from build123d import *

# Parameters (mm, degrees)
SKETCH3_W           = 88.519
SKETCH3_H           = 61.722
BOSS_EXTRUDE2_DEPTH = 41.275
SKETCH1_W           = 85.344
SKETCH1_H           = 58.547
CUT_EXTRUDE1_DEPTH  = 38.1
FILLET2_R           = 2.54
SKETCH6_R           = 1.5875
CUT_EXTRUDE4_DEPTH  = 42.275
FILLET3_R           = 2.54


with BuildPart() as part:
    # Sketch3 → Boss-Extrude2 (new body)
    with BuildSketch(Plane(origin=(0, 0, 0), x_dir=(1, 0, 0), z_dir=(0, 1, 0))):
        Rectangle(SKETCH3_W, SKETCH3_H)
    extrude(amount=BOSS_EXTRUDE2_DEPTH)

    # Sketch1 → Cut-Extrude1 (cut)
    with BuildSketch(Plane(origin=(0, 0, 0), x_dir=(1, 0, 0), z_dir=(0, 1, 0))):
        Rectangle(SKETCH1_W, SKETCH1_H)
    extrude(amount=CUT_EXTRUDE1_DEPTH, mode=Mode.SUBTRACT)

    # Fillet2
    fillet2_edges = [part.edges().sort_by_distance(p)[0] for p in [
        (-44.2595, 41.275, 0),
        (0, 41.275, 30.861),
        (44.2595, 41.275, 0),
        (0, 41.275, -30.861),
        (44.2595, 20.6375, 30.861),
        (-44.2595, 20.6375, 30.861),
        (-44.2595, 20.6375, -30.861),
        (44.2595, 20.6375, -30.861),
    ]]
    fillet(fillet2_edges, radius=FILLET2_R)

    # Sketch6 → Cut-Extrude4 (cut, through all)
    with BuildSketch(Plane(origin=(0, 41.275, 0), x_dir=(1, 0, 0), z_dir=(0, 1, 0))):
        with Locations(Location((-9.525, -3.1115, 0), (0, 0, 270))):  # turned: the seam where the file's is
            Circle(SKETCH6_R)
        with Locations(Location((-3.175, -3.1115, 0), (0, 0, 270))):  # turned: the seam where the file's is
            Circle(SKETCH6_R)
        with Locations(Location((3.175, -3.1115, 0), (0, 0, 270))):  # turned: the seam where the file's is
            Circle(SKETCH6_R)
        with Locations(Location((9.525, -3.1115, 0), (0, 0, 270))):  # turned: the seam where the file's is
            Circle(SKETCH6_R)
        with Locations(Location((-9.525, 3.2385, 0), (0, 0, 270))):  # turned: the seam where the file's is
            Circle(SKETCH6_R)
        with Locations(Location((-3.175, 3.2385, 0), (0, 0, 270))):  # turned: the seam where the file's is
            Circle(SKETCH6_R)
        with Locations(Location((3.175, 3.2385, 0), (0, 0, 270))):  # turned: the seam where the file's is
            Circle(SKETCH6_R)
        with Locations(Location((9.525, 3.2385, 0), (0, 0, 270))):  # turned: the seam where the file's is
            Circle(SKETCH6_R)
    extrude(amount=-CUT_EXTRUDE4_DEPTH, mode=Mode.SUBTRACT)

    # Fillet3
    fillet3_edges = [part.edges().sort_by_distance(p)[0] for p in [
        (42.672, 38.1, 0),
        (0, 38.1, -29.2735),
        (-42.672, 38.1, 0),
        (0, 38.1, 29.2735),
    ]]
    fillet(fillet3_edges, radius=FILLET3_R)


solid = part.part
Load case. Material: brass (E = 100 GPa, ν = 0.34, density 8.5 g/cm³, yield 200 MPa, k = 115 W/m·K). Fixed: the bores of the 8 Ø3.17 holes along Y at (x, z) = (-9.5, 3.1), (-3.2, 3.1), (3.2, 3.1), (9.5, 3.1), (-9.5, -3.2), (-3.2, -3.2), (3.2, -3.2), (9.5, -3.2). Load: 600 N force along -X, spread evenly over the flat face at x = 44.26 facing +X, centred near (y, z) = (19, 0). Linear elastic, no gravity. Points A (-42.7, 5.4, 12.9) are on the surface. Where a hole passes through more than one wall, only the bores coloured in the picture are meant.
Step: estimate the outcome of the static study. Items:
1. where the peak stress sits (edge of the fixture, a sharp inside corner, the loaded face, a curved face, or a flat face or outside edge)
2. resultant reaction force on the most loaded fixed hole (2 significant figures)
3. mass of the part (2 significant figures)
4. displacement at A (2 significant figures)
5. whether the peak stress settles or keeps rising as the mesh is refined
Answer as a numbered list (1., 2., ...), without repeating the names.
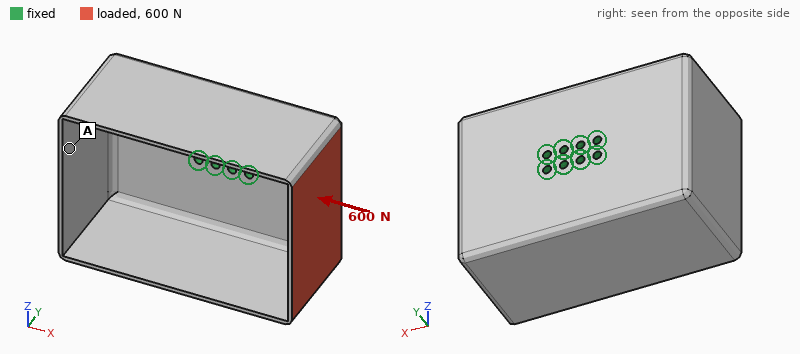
1. edge of the fixture
2. 250 N
3. 290 g
4. 0.13 mm
5. keeps rising
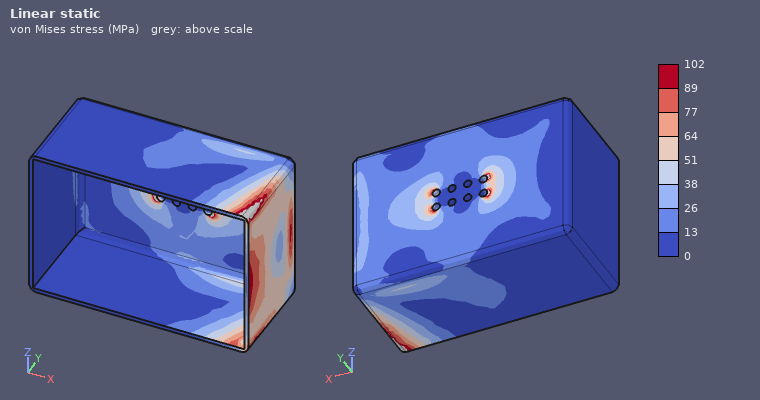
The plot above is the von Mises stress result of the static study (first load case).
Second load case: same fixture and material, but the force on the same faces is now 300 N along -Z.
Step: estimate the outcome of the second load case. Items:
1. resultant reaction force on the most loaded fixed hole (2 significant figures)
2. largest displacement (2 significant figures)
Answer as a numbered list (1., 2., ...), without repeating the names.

1. 430 N
2. 0.23 mm
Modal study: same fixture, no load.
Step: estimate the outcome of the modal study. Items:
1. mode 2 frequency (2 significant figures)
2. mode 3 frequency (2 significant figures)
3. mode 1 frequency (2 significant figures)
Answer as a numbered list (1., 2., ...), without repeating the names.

1. 640 Hz
2. 640 Hz
3. 610 Hz
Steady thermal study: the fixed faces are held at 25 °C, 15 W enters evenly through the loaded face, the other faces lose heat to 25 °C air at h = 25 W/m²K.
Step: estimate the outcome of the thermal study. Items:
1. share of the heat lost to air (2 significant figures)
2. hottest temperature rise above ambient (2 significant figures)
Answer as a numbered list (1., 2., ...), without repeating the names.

1. 36 %
2. 29 K
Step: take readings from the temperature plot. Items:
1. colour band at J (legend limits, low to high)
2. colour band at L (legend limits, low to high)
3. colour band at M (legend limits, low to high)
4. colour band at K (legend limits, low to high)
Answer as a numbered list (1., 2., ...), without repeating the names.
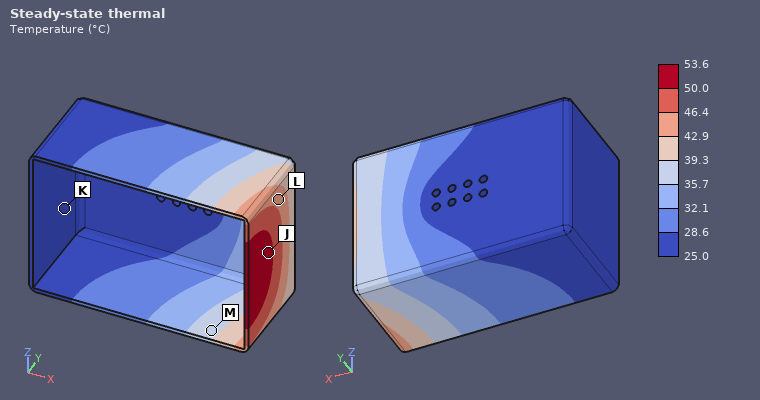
1. 50.0 to 53.6 °C
2. 42.9 to 46.4 °C
3. 35.7 to 39.3 °C
4. 25.0 to 28.6 °C
